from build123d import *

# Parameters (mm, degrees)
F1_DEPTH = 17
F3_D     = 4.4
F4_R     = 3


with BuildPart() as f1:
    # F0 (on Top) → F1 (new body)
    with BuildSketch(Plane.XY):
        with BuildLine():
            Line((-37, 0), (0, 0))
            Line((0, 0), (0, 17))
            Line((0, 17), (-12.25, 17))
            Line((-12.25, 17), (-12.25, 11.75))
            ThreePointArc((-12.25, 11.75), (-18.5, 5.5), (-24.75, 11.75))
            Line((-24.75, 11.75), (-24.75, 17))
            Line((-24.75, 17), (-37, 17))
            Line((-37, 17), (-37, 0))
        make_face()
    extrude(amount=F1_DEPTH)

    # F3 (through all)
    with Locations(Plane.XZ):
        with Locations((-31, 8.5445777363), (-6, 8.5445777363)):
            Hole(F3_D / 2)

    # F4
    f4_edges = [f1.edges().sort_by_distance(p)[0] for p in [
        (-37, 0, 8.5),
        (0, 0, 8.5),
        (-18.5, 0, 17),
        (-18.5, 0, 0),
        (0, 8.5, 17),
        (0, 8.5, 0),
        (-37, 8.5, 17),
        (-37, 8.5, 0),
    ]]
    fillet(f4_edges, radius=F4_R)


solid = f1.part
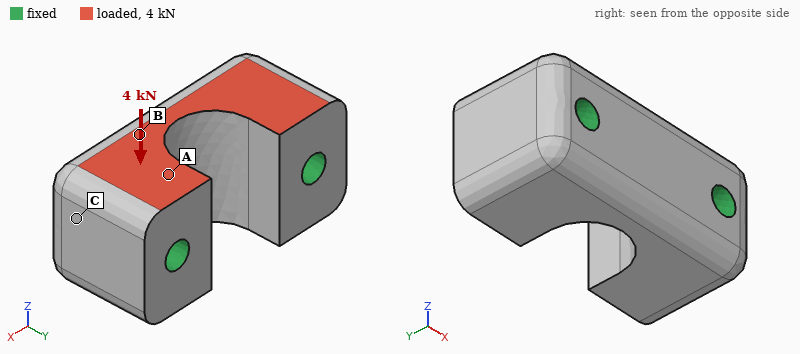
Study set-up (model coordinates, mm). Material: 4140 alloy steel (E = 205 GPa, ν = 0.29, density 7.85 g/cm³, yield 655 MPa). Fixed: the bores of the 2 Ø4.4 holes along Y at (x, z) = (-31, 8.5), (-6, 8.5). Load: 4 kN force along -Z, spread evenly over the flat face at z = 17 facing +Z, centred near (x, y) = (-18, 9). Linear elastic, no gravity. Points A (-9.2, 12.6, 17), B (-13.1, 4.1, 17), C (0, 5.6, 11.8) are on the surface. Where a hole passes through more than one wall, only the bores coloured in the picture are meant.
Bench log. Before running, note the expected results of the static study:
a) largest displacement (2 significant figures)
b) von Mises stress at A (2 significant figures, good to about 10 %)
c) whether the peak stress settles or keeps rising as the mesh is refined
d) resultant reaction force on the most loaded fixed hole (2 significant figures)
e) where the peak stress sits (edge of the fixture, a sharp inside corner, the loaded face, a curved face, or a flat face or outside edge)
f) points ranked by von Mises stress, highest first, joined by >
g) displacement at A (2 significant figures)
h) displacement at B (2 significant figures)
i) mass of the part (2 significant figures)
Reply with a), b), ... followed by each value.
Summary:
a) 1.0 µm
b) 13 MPa
c) keeps rising
d) 2.0 kN
e) edge of the fixture
f) A > B > C
g) 0.79 µm
h) 0.77 µm
i) 60 g
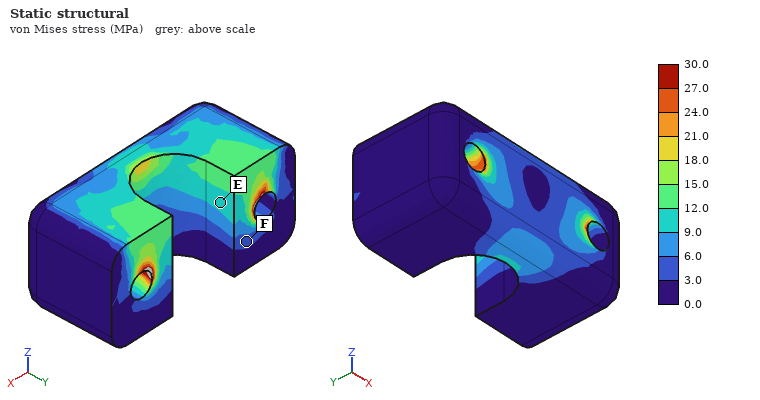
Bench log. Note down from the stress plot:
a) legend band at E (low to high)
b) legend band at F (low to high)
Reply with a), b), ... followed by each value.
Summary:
a) 9.0 to 12.0 MPa
b) 3.0 to 6.0 MPa
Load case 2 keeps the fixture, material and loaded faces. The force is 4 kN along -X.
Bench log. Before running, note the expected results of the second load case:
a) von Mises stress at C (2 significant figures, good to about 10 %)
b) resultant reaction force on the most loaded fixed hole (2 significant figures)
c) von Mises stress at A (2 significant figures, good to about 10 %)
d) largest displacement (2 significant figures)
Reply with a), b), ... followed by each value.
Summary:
a) 15 MPa
b) 2.1 kN
c) 29 MPa
d) 2.9 µm
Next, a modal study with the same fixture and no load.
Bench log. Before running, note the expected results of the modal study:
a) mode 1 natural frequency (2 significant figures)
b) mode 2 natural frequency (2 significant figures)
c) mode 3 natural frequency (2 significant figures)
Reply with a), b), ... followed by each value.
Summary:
a) 49 kHz
b) 62 kHz
c) 64 kHz
